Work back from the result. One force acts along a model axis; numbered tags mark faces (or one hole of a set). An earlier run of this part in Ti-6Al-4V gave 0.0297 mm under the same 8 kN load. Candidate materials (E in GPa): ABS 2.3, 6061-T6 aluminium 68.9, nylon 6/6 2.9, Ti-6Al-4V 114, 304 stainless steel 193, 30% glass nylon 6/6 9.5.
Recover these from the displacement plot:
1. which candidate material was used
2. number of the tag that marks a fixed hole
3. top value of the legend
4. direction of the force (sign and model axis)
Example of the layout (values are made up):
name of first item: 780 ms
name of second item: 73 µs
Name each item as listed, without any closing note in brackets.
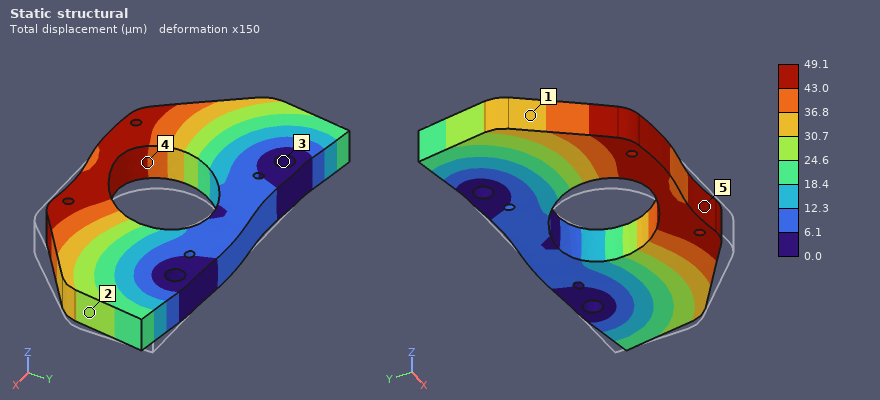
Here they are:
which candidate material was used: 6061-T6 aluminium
number of the tag that marks a fixed hole: 3
top value of the legend: 49.1 µm
direction of the force: -X
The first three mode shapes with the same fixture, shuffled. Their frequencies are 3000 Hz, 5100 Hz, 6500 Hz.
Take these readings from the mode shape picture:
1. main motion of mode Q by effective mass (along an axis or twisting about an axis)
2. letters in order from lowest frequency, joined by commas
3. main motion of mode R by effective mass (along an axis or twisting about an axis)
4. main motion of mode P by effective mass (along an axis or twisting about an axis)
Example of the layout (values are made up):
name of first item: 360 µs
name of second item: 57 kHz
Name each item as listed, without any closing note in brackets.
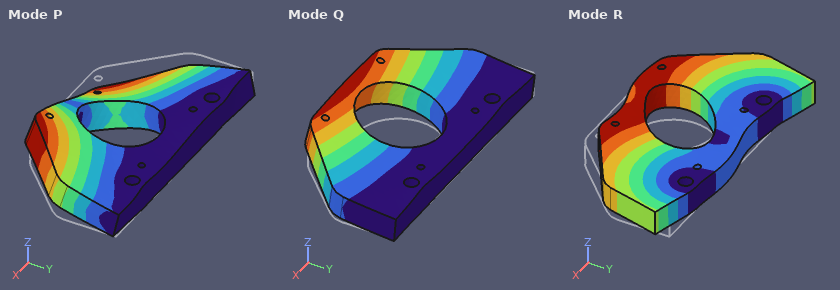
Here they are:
main motion of mode Q by effective mass: along Z
letters in order from lowest frequency, joined by commas: Q, P, R
main motion of mode R by effective mass: along X
main motion of mode P by effective mass: twisting about Y
